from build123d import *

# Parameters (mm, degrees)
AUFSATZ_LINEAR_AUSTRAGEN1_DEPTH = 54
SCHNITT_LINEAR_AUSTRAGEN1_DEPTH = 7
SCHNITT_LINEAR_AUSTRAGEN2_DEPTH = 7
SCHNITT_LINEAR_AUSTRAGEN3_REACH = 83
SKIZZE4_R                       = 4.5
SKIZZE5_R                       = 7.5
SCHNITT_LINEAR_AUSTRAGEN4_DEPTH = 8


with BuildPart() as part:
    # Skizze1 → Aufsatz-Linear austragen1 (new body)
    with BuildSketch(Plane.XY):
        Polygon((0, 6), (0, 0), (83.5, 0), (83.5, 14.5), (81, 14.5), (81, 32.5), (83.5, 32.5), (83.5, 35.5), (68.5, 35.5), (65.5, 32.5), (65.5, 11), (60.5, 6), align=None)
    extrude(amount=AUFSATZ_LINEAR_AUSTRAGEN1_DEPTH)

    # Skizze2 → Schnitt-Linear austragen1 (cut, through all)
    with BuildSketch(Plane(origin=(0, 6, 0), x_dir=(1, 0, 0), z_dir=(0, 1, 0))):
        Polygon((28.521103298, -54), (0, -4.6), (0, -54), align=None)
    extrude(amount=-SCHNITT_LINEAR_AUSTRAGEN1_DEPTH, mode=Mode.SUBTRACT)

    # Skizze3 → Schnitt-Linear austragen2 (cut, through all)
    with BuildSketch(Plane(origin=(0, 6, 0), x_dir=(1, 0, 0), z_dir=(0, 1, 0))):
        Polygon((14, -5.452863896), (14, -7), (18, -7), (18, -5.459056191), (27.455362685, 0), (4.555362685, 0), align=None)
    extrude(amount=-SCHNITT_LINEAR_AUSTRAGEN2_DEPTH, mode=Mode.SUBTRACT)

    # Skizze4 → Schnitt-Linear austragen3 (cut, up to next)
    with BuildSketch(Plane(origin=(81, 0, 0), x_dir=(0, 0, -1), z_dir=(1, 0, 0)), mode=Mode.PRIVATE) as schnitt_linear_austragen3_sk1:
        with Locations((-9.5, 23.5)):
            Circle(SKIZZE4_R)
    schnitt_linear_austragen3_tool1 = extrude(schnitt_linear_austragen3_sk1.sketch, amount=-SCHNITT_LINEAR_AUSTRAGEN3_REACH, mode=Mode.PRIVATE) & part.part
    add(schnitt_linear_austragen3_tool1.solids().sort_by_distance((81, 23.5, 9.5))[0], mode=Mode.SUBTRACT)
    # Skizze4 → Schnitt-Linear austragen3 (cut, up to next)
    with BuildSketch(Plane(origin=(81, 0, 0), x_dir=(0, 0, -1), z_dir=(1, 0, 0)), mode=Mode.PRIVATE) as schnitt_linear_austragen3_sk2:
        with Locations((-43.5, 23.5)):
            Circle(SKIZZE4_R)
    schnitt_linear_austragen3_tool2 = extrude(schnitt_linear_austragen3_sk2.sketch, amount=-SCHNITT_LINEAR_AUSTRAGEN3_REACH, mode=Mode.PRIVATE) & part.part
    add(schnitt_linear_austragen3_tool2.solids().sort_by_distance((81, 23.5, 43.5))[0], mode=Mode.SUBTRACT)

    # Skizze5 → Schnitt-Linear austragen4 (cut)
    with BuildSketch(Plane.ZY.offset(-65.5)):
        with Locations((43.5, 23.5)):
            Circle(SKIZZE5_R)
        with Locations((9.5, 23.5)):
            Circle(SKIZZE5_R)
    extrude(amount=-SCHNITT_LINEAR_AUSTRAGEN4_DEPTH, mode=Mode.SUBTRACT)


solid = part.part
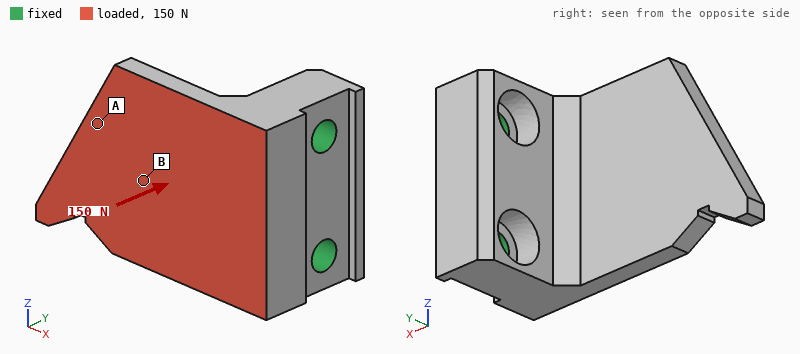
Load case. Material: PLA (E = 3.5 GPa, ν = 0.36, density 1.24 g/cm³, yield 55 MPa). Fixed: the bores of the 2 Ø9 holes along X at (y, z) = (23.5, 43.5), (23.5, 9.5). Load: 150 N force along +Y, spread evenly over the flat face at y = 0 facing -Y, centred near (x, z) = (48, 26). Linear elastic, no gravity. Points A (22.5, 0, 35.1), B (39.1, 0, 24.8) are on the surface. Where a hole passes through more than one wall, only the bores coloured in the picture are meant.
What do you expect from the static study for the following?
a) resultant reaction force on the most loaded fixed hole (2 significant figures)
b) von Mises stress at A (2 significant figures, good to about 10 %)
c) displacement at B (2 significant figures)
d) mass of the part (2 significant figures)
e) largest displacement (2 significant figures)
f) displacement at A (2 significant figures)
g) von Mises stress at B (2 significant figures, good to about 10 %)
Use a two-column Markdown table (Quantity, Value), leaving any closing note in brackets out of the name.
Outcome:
| Quantity | Value |
|---|---|
| resultant reaction force on the most loaded fixed hole | 81 N |
| von Mises stress at A | 1.2 MPa |
| displacement at B | 0.30 mm |
| mass of the part | 56 g |
| largest displacement | 0.98 mm |
| displacement at A | 0.53 mm |
| von Mises stress at B | 2.2 MPa |
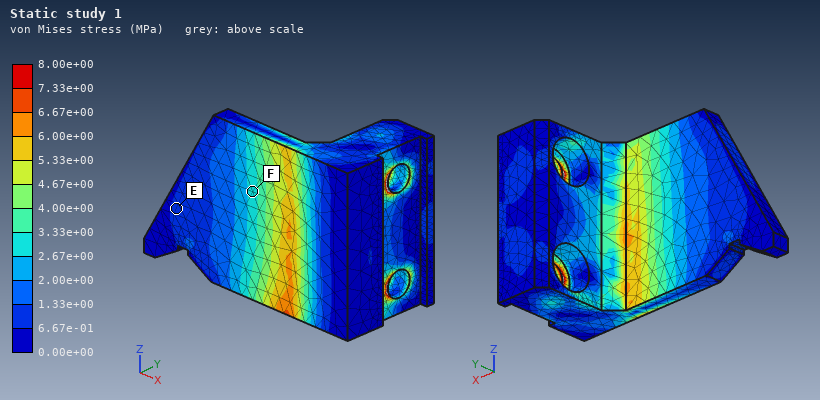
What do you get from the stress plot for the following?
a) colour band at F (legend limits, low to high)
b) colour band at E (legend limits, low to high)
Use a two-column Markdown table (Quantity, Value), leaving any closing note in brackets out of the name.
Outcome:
| Quantity | Value |
|---|---|
| colour band at F | 2.67e+00 to 3.33e+00 MPa |
| colour band at E | 6.67e-01 to 1.33e+00 MPa |
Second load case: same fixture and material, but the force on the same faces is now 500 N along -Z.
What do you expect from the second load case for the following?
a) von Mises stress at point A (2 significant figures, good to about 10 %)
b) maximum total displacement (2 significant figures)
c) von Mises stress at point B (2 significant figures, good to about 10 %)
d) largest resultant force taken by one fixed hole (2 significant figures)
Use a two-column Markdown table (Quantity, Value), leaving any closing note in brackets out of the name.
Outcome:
| Quantity | Value |
|---|---|
| von Mises stress at point A | 1.4 MPa |
| maximum total displacement | 0.26 mm |
| von Mises stress at point B | 2.5 MPa |
| largest resultant force taken by one fixed hole | 550 N |
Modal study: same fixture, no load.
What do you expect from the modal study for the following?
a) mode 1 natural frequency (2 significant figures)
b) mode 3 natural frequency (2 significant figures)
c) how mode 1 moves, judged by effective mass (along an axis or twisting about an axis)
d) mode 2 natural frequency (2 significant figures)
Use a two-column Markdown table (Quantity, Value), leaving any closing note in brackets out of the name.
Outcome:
| Quantity | Value |
|---|---|
| mode 1 natural frequency | 530 Hz |
| mode 3 natural frequency | 1700 Hz |
| how mode 1 moves, judged by effective mass | along Y |
| mode 2 natural frequency | 1400 Hz |
